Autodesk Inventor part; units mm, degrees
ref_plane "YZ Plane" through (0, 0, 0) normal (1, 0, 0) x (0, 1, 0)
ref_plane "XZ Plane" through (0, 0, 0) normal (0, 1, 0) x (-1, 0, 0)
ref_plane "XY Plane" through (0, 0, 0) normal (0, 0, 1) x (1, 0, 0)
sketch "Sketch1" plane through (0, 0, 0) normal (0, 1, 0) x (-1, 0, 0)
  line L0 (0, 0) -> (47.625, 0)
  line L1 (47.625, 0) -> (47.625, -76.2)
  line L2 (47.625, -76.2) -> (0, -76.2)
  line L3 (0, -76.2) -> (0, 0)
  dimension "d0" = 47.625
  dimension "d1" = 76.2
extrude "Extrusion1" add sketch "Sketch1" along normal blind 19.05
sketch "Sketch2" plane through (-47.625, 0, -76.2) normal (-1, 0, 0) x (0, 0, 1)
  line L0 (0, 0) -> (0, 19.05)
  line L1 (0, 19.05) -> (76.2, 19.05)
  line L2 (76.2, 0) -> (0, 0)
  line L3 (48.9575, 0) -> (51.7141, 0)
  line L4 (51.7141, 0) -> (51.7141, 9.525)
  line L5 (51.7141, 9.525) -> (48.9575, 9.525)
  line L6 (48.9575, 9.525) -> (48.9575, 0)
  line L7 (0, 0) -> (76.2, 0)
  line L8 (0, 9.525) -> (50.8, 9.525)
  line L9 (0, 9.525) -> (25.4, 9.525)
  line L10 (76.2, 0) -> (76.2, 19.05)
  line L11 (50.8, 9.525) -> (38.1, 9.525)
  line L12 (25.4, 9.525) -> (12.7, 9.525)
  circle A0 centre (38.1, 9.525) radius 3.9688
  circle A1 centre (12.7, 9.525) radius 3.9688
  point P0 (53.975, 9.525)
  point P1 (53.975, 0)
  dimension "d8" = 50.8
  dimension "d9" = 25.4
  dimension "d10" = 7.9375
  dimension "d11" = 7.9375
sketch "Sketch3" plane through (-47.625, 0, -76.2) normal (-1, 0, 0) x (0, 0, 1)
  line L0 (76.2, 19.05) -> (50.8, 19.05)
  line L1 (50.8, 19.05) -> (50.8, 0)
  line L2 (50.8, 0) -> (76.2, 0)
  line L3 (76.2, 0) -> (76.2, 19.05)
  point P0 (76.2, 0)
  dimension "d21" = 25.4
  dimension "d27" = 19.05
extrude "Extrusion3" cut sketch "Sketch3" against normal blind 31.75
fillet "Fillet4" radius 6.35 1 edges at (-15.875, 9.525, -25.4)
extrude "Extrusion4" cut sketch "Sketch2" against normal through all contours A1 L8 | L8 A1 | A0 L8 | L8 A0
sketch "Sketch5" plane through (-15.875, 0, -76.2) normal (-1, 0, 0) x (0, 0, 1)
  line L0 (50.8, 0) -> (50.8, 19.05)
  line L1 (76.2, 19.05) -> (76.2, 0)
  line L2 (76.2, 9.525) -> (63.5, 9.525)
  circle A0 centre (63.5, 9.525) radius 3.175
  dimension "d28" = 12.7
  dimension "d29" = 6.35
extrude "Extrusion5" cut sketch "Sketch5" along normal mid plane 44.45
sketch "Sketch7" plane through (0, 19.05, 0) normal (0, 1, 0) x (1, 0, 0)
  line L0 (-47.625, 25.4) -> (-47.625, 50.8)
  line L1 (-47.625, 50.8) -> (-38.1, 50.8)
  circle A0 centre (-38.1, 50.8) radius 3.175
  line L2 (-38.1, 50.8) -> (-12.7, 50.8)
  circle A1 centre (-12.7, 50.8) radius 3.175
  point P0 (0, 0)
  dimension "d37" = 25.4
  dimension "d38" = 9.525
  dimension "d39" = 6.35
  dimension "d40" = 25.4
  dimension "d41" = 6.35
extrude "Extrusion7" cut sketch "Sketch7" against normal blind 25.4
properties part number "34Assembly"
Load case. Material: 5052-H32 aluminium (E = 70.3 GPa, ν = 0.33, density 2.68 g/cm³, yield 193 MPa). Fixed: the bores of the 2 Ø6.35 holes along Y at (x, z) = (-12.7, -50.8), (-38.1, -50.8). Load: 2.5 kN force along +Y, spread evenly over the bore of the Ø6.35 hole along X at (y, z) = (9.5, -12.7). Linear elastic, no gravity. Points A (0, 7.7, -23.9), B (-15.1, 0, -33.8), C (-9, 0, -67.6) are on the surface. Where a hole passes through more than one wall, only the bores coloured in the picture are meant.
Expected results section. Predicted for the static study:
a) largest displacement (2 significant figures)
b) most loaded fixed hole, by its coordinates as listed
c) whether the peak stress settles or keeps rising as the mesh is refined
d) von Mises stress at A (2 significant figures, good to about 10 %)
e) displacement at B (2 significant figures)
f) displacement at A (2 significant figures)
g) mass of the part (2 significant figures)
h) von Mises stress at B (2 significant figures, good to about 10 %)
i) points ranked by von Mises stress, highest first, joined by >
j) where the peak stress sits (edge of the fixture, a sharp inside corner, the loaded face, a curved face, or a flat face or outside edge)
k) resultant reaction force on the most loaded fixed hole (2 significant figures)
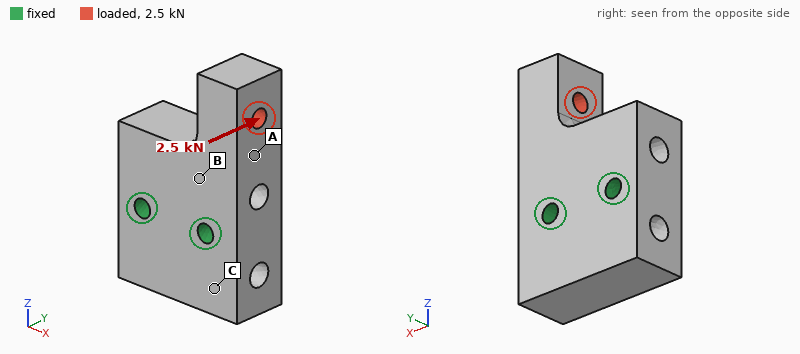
85 µm
(-12.7, -50.8)
keeps rising
20 MPa
19 µm
35 µm
130 g
35 MPa
B > A > C
edge of the fixture
2.2 kN
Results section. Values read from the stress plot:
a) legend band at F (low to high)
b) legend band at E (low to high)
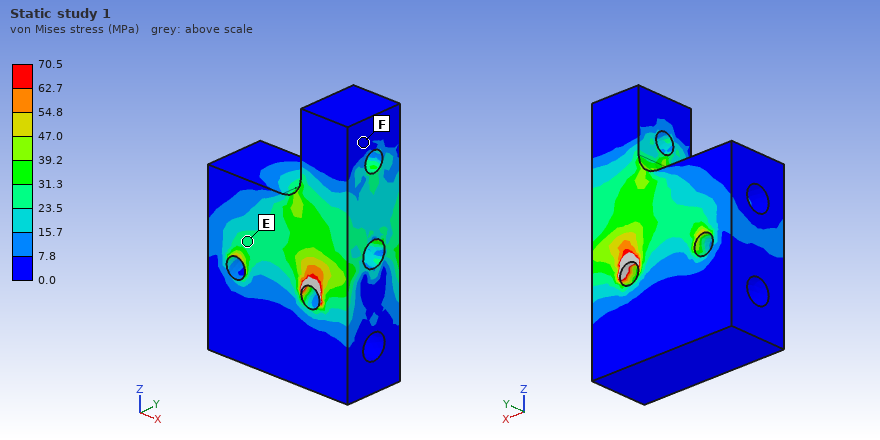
0.0 to 7.8 MPa
23.5 to 31.3 MPa
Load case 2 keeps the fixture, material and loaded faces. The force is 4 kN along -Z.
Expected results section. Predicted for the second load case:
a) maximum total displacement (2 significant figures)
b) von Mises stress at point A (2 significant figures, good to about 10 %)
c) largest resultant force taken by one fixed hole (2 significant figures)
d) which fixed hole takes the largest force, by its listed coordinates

18 µm
13 MPa
4.4 kN
(-12.7, -50.8)
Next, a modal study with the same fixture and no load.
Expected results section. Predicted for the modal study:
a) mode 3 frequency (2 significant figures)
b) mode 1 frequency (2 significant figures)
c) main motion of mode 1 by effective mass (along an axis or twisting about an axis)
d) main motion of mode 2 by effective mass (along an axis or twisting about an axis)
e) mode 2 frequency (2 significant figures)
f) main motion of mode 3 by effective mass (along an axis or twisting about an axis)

16 kHz
6800 Hz
along Y
along X
9200 Hz
along Y
